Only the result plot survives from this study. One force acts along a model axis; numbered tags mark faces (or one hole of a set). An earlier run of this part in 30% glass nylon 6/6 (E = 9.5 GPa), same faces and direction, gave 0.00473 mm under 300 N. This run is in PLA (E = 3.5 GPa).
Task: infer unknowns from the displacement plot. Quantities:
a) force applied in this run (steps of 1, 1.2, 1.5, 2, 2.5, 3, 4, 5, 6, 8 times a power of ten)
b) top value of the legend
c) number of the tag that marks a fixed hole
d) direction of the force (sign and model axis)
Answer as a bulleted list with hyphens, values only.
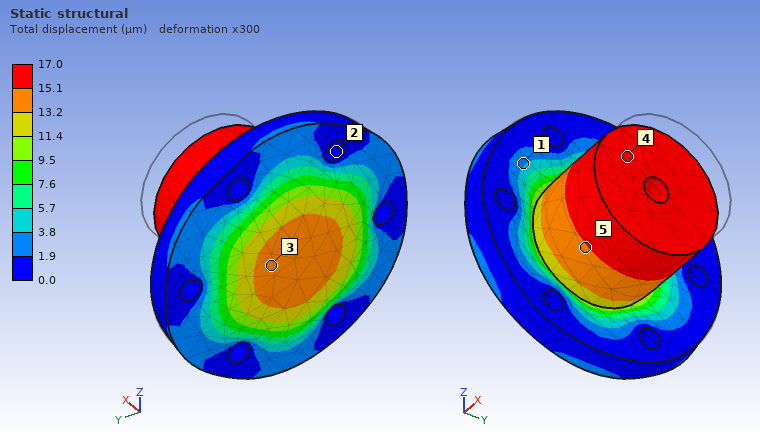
- 400 N
- 17.0 µm
- 2
- -X
